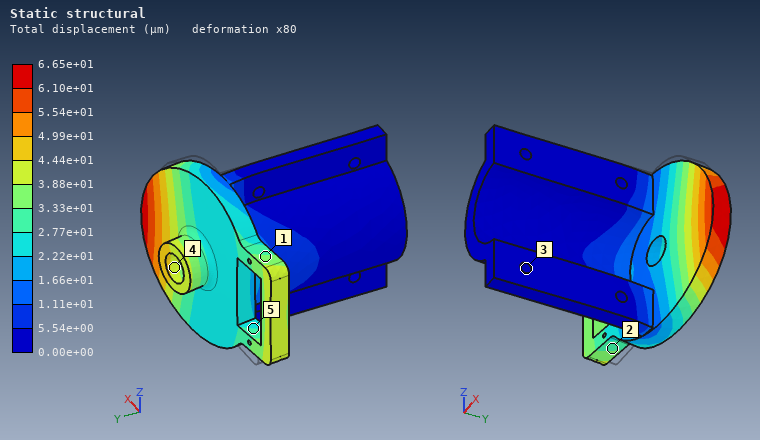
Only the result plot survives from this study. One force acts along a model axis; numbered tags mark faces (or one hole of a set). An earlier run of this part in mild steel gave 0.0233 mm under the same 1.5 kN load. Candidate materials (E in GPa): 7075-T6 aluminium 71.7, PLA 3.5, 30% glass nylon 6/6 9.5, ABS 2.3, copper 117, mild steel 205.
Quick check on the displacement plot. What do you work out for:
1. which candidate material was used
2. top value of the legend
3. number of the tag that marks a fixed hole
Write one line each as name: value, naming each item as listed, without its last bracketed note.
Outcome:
which candidate material was used: 7075-T6 aluminium
top value of the legend: 6.65e+01 µm
number of the tag that marks a fixed hole: 3
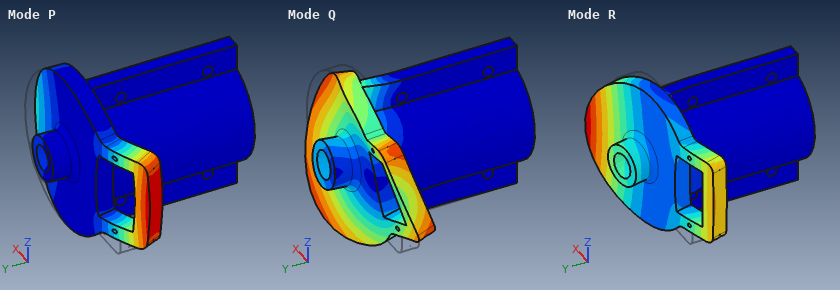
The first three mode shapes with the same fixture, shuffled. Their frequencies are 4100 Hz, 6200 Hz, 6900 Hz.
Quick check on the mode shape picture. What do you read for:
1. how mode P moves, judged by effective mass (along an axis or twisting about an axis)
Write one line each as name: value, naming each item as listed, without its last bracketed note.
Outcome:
how mode P moves, judged by effective mass: along Y
